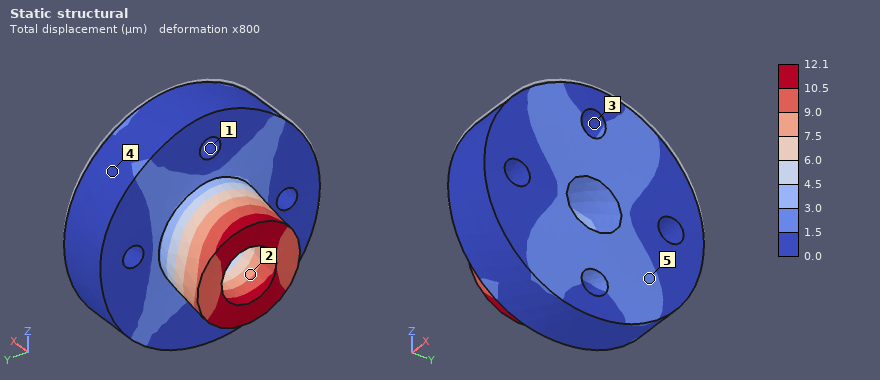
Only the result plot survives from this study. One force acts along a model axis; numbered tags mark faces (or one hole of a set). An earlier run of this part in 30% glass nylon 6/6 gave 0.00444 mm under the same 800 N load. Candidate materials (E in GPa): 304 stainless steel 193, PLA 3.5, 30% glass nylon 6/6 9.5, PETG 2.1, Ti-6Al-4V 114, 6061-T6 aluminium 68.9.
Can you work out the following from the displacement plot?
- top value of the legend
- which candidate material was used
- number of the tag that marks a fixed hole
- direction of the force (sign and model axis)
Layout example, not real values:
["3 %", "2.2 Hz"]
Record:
["12.1 µm", "PLA", "1", "-Z"]
